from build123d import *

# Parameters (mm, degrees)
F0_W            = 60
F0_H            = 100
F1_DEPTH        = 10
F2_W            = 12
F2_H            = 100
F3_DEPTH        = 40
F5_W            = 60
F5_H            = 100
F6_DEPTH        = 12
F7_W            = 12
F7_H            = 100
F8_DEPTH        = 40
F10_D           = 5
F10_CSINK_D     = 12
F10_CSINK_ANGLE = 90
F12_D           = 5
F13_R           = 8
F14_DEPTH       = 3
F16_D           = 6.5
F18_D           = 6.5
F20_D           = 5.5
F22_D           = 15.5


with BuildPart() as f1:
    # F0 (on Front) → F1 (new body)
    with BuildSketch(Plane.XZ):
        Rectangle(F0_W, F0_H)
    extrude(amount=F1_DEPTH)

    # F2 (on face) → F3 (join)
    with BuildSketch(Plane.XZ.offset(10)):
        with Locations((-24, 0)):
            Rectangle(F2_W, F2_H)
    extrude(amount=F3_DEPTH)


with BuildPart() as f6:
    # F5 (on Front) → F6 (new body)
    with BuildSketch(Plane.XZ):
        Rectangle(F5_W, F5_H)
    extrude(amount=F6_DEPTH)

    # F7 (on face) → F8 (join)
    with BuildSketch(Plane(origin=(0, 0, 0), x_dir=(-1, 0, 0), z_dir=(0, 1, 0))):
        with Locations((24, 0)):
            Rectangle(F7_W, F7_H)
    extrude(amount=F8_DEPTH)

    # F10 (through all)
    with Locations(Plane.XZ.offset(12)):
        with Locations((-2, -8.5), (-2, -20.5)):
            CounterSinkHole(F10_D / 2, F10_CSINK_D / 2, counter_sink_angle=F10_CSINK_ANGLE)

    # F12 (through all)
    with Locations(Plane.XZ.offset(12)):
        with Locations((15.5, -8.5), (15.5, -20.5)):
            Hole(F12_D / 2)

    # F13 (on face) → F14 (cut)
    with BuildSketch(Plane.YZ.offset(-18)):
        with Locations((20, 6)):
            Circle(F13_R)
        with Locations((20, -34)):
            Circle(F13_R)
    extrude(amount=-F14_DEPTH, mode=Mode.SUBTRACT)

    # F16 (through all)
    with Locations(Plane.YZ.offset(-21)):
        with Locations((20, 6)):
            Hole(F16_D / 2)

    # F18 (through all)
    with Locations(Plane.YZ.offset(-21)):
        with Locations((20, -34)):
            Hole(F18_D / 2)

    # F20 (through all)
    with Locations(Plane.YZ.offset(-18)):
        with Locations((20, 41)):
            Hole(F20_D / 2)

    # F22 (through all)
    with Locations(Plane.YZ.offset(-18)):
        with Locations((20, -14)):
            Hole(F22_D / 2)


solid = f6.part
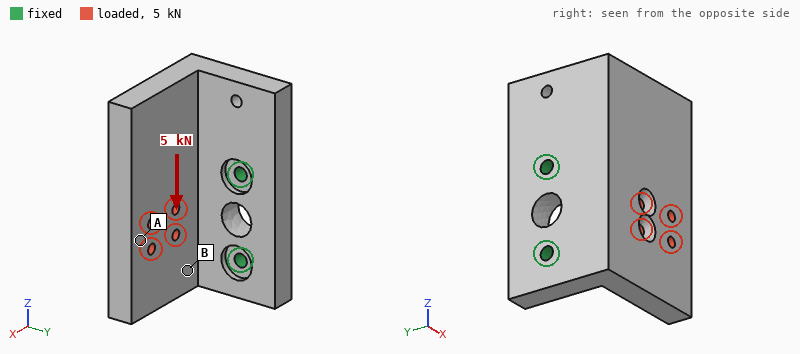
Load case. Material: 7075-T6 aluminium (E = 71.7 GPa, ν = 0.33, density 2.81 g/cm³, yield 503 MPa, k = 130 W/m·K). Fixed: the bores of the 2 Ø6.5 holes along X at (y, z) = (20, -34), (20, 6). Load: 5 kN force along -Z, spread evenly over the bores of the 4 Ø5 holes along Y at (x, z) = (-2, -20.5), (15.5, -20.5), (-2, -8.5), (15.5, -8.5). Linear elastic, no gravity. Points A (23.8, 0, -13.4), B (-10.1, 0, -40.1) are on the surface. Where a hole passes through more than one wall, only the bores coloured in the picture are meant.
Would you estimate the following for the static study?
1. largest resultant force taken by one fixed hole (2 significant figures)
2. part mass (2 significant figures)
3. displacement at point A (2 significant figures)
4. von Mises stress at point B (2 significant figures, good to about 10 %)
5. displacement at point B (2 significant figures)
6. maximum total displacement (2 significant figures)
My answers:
5.1 kN
320 g
0.100 mm
32 MPa
0.054 mm
0.16 mm
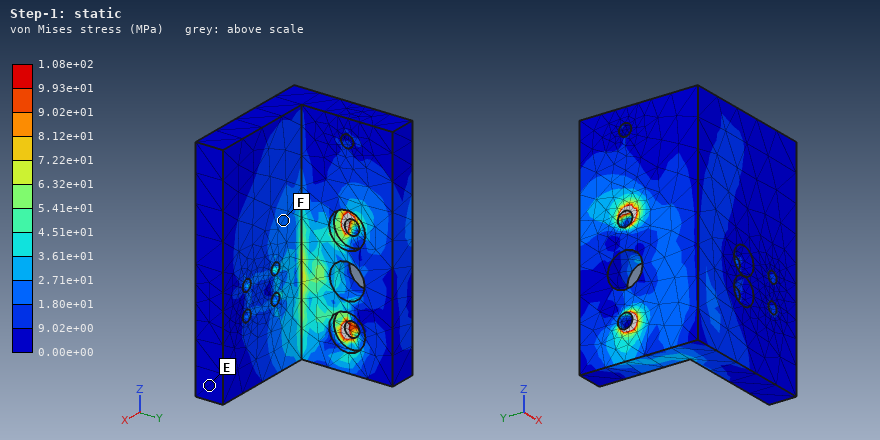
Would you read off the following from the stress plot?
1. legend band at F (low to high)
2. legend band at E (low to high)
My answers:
1.80e+01 to 2.71e+01 MPa
0.00e+00 to 9.02e+00 MPa
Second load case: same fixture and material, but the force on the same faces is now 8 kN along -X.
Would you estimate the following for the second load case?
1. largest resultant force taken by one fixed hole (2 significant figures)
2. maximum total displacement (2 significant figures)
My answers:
4.1 kN
0.37 mm
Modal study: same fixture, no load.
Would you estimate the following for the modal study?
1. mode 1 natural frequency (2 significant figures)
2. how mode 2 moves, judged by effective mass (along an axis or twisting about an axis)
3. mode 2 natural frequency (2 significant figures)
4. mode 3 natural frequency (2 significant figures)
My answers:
1400 Hz
along Z
2400 Hz
3800 Hz
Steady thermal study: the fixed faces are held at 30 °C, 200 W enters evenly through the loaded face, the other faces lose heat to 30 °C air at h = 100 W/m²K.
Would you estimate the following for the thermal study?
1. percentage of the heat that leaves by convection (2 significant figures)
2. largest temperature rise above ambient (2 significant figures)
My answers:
40 %
83 K
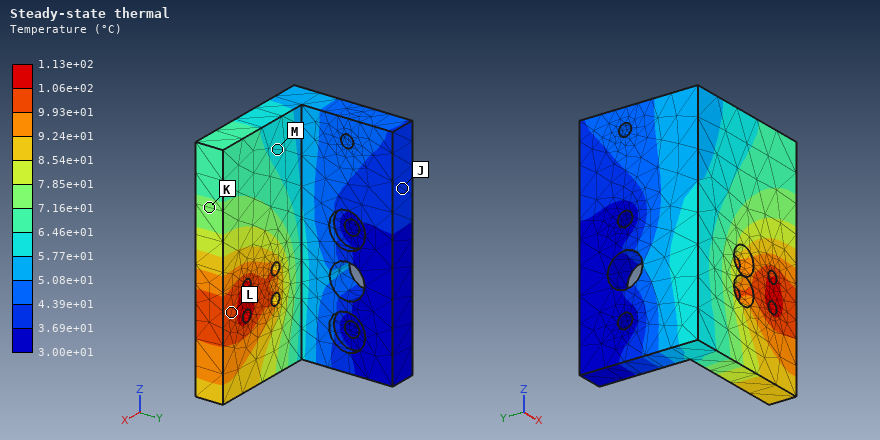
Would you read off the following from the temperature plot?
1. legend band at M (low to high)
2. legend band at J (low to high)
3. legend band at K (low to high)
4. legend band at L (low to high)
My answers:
5.77e+01 to 6.46e+01 °C
3.69e+01 to 4.39e+01 °C
7.16e+01 to 7.85e+01 °C
9.93e+01 to 1.06e+02 °C
